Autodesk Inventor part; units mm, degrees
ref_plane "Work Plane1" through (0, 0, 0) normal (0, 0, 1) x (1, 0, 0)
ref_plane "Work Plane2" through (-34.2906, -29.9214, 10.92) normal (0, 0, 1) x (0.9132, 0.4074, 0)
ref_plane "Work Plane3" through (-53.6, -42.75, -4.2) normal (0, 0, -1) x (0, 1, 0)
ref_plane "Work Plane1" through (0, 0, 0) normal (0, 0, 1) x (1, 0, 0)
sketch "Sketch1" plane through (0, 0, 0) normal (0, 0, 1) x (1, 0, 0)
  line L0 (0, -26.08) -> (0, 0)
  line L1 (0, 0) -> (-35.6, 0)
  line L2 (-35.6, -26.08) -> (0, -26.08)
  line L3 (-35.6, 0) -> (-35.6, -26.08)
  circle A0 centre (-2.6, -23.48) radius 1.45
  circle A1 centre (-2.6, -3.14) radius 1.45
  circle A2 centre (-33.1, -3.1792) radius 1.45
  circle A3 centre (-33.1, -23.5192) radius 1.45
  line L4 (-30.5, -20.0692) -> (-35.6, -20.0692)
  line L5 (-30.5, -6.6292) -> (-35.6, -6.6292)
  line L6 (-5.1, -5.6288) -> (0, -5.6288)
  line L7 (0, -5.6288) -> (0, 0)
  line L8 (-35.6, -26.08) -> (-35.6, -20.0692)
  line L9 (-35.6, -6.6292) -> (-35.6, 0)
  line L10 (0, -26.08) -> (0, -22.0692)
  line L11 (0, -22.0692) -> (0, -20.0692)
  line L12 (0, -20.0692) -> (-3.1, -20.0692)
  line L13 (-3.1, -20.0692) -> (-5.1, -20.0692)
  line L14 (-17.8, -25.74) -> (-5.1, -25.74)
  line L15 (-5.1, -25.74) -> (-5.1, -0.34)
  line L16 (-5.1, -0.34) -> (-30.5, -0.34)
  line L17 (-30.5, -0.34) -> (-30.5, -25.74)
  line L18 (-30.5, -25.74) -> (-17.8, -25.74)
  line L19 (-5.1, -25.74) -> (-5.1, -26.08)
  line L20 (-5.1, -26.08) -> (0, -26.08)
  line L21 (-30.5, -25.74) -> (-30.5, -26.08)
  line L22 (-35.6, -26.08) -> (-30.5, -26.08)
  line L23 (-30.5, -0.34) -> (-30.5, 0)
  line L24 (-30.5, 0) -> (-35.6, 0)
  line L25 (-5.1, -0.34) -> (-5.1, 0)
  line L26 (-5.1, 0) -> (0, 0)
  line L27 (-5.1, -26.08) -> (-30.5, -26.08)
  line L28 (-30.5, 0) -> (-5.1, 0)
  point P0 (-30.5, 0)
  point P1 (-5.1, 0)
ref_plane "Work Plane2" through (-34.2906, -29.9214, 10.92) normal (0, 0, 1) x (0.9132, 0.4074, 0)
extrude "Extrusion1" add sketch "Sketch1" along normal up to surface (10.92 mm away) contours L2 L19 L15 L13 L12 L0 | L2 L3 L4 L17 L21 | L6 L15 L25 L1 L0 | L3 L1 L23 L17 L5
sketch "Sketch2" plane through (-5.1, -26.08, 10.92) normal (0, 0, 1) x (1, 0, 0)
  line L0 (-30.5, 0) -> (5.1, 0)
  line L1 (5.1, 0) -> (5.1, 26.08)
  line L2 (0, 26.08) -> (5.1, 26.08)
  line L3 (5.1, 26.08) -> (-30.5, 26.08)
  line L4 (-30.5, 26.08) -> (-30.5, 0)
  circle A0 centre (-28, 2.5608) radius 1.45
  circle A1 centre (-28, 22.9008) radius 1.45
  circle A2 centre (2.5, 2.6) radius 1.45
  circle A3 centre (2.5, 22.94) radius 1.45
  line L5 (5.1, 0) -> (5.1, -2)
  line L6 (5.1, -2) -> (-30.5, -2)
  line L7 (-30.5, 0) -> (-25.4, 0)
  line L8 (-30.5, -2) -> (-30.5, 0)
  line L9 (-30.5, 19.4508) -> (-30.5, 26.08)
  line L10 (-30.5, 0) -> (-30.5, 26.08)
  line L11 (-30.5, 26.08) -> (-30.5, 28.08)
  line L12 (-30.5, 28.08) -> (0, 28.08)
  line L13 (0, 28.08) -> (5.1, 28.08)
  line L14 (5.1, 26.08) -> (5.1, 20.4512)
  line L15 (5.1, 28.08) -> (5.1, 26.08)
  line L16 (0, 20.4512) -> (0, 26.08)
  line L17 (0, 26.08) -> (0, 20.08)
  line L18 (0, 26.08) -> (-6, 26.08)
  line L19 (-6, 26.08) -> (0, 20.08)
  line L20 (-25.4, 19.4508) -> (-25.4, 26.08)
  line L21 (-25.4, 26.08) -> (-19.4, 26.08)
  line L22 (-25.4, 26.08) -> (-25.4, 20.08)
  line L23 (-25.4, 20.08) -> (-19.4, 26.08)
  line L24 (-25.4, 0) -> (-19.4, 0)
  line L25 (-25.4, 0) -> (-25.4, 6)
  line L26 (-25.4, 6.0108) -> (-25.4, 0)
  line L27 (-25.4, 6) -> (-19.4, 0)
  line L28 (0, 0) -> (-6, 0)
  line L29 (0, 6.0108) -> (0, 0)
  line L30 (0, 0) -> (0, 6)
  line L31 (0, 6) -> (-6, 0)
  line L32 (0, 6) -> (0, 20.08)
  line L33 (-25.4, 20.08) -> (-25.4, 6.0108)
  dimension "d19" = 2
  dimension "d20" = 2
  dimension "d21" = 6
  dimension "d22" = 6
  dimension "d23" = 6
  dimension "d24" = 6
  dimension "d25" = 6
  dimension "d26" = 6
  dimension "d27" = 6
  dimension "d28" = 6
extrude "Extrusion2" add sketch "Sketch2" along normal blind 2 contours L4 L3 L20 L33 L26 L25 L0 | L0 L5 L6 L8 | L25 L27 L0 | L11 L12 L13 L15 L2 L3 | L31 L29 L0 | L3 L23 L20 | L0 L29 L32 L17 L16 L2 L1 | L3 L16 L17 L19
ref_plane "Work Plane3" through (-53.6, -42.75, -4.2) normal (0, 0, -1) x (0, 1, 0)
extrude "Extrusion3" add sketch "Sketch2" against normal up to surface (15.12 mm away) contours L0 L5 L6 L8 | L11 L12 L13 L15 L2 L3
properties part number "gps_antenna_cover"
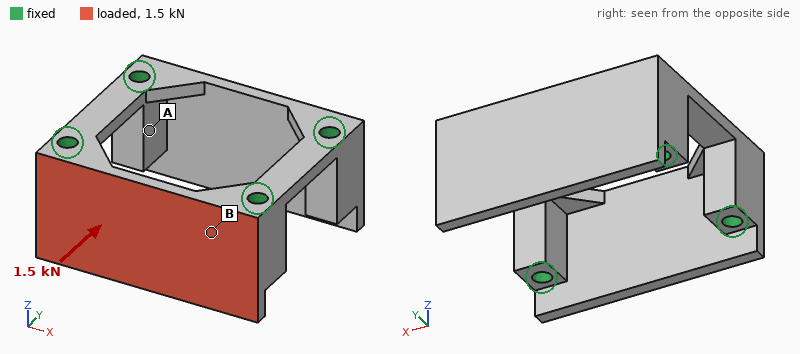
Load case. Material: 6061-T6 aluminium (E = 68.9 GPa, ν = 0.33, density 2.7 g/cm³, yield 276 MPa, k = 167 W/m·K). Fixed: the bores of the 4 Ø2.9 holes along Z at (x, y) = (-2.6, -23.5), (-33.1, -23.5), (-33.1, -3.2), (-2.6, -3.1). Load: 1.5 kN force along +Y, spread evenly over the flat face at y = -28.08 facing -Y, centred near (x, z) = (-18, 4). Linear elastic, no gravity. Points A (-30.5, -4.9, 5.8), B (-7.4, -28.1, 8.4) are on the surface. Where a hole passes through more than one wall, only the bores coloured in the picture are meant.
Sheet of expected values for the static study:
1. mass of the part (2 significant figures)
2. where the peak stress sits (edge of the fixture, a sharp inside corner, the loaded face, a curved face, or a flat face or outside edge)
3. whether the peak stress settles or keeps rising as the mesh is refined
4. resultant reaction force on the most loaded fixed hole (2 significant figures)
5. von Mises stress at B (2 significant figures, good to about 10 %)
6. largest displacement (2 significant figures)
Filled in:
11 g
a sharp inside corner
keeps rising
830 N
67 MPa
0.11 mm
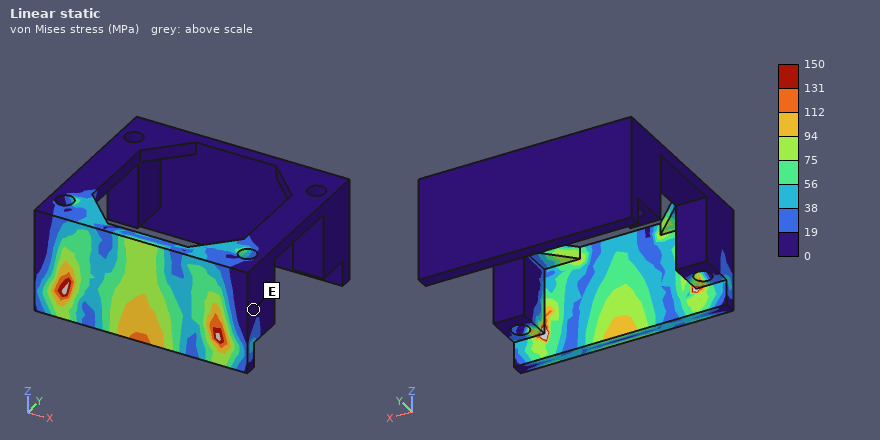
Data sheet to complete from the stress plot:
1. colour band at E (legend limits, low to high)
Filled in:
0 to 19 MPa
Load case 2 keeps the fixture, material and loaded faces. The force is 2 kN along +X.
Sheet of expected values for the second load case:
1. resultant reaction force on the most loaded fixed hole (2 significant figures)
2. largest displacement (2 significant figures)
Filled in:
1.0 kN
7.8 µm
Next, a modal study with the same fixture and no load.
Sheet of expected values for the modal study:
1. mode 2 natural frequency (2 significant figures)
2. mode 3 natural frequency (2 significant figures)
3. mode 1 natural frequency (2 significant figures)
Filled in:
14 kHz
25 kHz
14 kHz
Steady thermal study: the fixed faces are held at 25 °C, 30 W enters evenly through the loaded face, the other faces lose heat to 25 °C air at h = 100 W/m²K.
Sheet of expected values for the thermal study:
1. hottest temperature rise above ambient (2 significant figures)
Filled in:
17 K
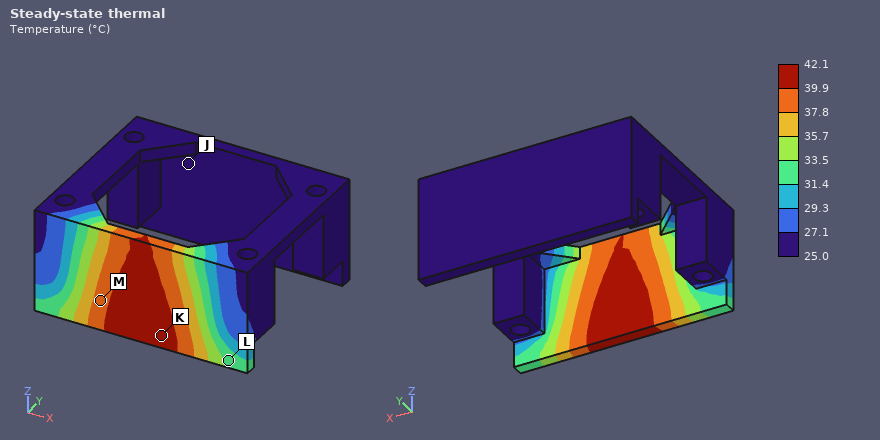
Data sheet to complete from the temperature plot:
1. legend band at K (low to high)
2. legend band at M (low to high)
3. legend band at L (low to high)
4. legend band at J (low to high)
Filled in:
39.9 to 42.1 °C
37.8 to 39.9 °C
31.4 to 33.5 °C
25.0 to 27.1 °C
